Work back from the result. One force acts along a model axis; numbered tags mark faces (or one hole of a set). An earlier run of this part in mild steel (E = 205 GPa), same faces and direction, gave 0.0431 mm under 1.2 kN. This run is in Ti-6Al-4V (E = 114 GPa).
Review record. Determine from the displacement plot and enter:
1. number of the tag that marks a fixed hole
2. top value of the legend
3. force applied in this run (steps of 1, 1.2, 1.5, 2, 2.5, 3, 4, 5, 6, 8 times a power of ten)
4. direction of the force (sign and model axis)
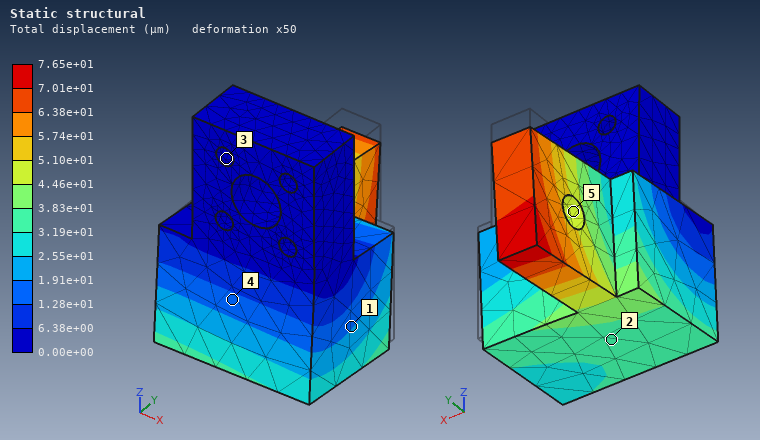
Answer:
3
7.65e+01 µm
1.2 kN
-Z
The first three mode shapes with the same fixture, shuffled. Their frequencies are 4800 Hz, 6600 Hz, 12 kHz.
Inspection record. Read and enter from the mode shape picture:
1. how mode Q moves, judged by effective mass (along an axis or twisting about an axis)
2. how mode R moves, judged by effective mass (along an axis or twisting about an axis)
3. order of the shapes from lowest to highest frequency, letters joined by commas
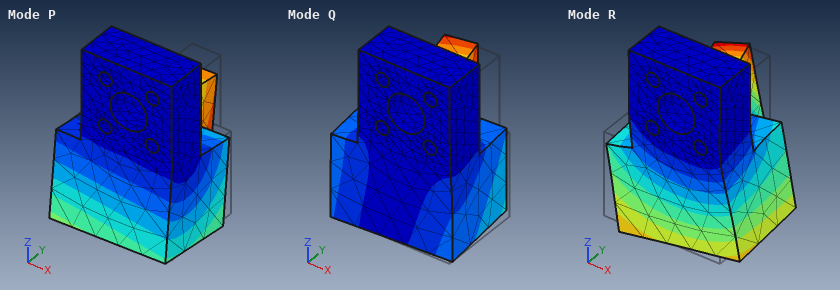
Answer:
along X
along X
P, Q, R
